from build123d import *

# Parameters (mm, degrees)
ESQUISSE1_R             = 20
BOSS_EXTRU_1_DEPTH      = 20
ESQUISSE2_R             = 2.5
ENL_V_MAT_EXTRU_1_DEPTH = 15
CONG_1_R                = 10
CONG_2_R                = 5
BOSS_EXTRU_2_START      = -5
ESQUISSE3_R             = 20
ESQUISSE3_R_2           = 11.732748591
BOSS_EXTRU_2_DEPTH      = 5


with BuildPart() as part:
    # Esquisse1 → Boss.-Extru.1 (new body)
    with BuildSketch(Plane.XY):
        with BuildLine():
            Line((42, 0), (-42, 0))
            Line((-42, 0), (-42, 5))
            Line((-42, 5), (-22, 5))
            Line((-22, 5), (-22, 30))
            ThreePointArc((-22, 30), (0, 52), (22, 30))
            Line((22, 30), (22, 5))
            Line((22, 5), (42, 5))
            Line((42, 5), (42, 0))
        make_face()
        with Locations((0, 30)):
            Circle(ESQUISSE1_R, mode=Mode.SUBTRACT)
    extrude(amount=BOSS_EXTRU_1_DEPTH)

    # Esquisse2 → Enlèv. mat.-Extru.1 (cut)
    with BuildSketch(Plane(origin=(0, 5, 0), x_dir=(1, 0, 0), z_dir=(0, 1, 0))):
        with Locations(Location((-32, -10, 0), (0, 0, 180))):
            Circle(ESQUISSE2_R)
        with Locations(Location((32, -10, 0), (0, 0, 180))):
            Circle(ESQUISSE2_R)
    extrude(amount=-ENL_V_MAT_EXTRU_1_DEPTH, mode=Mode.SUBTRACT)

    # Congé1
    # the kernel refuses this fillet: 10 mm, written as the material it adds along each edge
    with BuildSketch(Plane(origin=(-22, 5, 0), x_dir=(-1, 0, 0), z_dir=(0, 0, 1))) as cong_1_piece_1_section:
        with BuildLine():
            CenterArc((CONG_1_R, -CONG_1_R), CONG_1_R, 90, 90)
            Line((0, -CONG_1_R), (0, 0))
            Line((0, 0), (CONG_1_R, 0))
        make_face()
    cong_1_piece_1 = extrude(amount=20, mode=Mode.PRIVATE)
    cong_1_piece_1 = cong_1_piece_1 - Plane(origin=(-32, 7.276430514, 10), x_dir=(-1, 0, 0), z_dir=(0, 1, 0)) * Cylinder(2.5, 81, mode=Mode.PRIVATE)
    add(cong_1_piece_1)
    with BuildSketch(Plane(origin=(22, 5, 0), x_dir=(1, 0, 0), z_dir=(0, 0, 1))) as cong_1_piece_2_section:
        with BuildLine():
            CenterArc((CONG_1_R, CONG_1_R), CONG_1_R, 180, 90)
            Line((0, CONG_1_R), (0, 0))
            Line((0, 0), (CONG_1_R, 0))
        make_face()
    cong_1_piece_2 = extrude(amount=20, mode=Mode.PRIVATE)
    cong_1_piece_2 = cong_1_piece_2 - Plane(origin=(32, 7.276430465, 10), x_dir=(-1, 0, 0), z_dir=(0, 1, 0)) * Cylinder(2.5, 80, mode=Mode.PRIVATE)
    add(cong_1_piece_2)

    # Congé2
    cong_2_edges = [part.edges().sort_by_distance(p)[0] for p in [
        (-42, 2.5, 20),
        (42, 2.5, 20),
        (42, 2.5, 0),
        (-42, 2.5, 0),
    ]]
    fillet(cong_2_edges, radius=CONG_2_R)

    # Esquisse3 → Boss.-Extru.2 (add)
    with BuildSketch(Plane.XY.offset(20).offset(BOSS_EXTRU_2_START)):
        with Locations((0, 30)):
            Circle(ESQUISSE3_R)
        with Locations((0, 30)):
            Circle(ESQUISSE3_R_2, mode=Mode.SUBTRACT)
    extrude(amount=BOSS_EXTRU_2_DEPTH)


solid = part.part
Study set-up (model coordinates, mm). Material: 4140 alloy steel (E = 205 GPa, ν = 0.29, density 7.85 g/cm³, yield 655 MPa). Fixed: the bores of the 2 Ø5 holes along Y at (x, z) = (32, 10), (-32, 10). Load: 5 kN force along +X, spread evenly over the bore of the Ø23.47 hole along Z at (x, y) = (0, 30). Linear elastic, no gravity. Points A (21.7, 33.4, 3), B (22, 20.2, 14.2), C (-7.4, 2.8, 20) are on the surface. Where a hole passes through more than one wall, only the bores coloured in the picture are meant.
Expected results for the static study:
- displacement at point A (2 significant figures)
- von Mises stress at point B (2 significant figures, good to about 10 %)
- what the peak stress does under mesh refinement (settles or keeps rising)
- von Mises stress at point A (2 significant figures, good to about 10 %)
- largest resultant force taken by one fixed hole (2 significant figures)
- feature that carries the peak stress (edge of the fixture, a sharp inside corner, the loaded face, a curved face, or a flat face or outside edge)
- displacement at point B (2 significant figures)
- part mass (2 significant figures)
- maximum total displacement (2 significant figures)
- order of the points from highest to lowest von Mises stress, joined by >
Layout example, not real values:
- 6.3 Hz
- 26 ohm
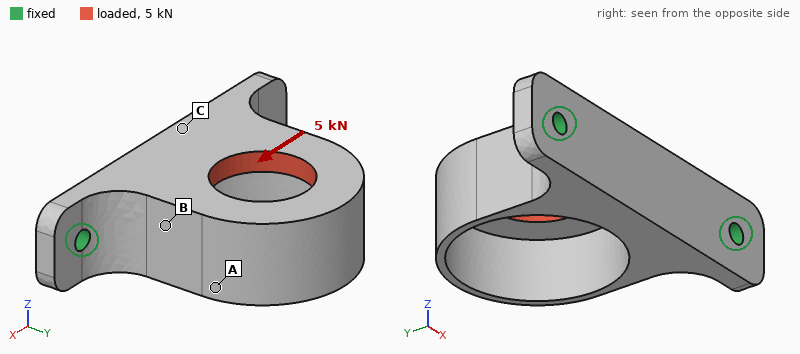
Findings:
- 29 µm
- 68 MPa
- keeps rising
- 29 MPa
- 3.5 kN
- edge of the fixture
- 12 µm
- 200 g
- 52 µm
- B > A > C
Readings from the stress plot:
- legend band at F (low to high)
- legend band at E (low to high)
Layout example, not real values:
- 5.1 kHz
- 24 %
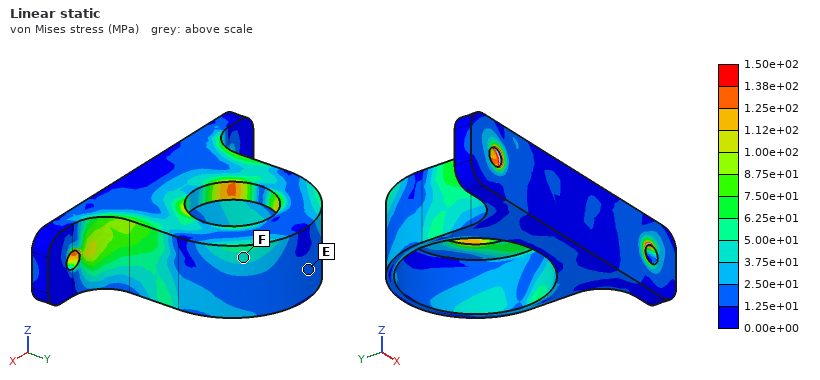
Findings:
- 3.75e+01 to 5.00e+01 MPa
- 1.25e+01 to 2.50e+01 MPa
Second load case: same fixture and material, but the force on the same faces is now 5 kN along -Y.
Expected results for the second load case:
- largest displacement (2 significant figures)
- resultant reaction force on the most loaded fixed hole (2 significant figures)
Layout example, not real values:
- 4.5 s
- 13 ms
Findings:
- 94 µm
- 3.2 kN
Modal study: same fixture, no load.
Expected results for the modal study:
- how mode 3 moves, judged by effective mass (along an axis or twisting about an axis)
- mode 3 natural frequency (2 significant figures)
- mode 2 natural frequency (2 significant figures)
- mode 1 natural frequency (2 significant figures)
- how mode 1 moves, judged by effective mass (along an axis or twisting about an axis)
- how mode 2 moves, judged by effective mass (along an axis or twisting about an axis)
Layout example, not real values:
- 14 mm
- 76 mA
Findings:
- along Y
- 8200 Hz
- 5700 Hz
- 2500 Hz
- along Z
- along X
